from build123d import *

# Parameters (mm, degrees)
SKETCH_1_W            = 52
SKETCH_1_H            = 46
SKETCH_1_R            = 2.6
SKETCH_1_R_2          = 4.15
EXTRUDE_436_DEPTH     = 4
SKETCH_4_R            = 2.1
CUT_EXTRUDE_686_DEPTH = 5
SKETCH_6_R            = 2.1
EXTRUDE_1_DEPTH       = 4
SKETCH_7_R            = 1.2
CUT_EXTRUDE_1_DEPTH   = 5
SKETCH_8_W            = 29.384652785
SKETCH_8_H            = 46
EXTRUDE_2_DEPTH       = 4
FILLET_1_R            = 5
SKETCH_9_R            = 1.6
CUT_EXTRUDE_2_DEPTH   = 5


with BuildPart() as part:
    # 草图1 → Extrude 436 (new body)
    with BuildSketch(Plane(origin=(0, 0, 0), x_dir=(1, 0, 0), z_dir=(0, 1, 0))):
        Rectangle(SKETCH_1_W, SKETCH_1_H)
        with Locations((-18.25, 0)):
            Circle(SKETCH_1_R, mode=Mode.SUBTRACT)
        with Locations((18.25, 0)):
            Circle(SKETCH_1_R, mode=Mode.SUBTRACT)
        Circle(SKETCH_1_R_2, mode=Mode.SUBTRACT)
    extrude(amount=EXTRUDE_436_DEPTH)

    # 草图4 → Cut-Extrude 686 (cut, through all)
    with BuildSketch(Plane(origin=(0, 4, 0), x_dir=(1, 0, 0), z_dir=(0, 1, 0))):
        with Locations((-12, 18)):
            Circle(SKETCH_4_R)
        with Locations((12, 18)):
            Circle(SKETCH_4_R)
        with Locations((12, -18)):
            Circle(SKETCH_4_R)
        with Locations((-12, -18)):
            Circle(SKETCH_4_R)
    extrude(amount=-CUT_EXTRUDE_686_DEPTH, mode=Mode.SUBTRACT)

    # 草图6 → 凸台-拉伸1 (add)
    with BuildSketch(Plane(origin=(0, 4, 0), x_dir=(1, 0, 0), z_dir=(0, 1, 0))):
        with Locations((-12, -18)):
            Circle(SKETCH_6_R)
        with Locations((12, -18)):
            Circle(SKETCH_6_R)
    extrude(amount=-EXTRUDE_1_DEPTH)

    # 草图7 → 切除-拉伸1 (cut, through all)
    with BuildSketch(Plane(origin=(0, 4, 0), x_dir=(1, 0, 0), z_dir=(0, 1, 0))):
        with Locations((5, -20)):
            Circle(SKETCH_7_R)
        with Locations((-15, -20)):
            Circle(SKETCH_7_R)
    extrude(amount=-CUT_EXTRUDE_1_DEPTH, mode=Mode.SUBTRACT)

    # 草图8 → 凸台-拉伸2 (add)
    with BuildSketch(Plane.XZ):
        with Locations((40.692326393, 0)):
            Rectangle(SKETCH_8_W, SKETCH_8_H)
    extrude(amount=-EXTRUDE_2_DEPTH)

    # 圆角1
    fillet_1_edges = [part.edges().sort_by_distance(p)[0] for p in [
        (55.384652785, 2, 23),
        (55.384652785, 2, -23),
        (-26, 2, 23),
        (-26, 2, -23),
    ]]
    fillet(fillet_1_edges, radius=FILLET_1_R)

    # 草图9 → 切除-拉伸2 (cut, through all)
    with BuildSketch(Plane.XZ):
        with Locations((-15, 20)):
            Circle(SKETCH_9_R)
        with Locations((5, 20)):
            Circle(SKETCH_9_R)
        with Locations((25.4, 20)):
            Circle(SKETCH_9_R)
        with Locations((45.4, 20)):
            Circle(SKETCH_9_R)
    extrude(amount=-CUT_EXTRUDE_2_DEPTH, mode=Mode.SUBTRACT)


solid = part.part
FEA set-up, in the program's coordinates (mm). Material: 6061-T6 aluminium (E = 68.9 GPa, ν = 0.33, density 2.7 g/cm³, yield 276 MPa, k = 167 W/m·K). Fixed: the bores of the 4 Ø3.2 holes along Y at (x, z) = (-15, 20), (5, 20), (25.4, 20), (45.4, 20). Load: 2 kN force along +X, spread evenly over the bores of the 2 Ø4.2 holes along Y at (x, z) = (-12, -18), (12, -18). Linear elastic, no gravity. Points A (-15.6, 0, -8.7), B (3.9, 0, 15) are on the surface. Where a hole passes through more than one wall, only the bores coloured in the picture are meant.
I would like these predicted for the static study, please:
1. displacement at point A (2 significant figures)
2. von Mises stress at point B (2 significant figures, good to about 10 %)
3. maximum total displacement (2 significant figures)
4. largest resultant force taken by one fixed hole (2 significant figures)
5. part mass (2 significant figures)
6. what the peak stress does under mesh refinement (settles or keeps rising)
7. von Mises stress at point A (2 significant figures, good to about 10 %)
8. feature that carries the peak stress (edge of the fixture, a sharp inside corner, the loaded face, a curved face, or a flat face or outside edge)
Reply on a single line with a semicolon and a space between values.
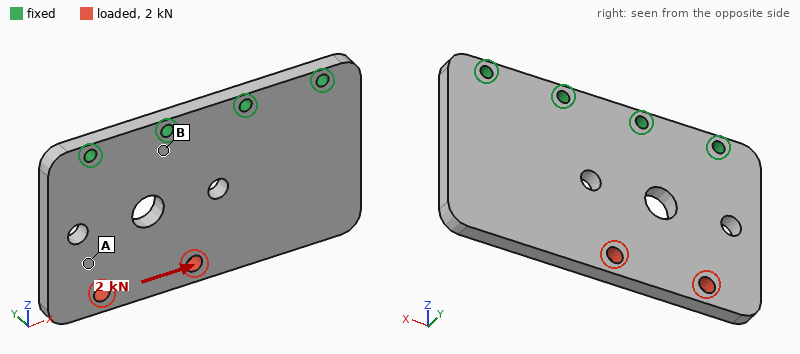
18 µm; 14 MPa; 27 µm; 1.2 kN; 39 g; keeps rising; 7.1 MPa; edge of the fixture
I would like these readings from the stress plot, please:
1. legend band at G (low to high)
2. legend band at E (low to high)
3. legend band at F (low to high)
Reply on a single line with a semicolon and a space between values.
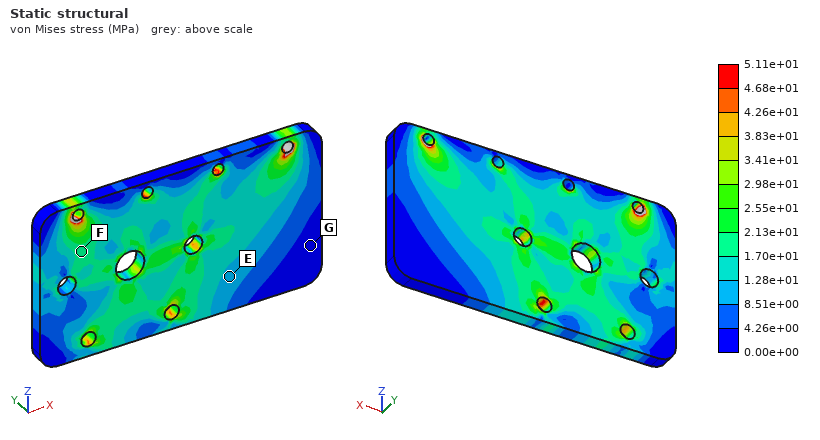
0.00e+00 to 4.26e+00 MPa; 8.51e+00 to 1.28e+01 MPa; 1.70e+01 to 2.13e+01 MPa
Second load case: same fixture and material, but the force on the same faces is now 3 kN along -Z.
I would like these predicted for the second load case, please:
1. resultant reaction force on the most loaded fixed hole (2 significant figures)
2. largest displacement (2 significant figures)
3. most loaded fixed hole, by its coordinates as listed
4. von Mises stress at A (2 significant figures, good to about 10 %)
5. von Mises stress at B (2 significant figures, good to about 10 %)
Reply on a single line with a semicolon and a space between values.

1.4 kN; 17 µm; (-15, 20); 19 MPa; 23 MPa
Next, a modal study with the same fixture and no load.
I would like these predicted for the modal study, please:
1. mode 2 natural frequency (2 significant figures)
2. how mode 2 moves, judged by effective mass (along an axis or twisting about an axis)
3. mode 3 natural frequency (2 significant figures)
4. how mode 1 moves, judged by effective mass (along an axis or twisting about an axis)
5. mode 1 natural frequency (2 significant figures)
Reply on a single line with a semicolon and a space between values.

2700 Hz; twisting about Z; 5200 Hz; along Y; 1700 Hz
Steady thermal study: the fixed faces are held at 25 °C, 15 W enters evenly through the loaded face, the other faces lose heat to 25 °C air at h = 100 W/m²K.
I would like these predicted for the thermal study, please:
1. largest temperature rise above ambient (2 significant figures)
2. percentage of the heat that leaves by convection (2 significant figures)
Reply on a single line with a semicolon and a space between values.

16 K; 28 %
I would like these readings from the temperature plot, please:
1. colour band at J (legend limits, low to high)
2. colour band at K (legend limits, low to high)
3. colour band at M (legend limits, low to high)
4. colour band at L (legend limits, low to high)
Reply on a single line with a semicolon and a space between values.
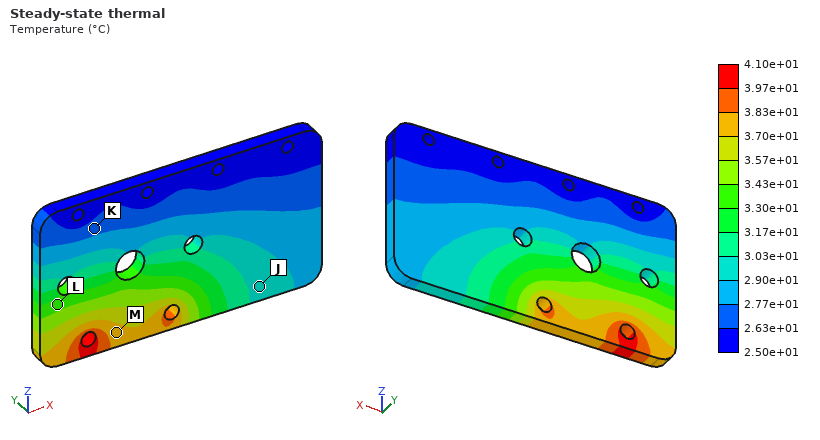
2.90e+01 to 3.03e+01 °C; 2.63e+01 to 2.77e+01 °C; 3.70e+01 to 3.83e+01 °C; 3.30e+01 to 3.43e+01 °C
